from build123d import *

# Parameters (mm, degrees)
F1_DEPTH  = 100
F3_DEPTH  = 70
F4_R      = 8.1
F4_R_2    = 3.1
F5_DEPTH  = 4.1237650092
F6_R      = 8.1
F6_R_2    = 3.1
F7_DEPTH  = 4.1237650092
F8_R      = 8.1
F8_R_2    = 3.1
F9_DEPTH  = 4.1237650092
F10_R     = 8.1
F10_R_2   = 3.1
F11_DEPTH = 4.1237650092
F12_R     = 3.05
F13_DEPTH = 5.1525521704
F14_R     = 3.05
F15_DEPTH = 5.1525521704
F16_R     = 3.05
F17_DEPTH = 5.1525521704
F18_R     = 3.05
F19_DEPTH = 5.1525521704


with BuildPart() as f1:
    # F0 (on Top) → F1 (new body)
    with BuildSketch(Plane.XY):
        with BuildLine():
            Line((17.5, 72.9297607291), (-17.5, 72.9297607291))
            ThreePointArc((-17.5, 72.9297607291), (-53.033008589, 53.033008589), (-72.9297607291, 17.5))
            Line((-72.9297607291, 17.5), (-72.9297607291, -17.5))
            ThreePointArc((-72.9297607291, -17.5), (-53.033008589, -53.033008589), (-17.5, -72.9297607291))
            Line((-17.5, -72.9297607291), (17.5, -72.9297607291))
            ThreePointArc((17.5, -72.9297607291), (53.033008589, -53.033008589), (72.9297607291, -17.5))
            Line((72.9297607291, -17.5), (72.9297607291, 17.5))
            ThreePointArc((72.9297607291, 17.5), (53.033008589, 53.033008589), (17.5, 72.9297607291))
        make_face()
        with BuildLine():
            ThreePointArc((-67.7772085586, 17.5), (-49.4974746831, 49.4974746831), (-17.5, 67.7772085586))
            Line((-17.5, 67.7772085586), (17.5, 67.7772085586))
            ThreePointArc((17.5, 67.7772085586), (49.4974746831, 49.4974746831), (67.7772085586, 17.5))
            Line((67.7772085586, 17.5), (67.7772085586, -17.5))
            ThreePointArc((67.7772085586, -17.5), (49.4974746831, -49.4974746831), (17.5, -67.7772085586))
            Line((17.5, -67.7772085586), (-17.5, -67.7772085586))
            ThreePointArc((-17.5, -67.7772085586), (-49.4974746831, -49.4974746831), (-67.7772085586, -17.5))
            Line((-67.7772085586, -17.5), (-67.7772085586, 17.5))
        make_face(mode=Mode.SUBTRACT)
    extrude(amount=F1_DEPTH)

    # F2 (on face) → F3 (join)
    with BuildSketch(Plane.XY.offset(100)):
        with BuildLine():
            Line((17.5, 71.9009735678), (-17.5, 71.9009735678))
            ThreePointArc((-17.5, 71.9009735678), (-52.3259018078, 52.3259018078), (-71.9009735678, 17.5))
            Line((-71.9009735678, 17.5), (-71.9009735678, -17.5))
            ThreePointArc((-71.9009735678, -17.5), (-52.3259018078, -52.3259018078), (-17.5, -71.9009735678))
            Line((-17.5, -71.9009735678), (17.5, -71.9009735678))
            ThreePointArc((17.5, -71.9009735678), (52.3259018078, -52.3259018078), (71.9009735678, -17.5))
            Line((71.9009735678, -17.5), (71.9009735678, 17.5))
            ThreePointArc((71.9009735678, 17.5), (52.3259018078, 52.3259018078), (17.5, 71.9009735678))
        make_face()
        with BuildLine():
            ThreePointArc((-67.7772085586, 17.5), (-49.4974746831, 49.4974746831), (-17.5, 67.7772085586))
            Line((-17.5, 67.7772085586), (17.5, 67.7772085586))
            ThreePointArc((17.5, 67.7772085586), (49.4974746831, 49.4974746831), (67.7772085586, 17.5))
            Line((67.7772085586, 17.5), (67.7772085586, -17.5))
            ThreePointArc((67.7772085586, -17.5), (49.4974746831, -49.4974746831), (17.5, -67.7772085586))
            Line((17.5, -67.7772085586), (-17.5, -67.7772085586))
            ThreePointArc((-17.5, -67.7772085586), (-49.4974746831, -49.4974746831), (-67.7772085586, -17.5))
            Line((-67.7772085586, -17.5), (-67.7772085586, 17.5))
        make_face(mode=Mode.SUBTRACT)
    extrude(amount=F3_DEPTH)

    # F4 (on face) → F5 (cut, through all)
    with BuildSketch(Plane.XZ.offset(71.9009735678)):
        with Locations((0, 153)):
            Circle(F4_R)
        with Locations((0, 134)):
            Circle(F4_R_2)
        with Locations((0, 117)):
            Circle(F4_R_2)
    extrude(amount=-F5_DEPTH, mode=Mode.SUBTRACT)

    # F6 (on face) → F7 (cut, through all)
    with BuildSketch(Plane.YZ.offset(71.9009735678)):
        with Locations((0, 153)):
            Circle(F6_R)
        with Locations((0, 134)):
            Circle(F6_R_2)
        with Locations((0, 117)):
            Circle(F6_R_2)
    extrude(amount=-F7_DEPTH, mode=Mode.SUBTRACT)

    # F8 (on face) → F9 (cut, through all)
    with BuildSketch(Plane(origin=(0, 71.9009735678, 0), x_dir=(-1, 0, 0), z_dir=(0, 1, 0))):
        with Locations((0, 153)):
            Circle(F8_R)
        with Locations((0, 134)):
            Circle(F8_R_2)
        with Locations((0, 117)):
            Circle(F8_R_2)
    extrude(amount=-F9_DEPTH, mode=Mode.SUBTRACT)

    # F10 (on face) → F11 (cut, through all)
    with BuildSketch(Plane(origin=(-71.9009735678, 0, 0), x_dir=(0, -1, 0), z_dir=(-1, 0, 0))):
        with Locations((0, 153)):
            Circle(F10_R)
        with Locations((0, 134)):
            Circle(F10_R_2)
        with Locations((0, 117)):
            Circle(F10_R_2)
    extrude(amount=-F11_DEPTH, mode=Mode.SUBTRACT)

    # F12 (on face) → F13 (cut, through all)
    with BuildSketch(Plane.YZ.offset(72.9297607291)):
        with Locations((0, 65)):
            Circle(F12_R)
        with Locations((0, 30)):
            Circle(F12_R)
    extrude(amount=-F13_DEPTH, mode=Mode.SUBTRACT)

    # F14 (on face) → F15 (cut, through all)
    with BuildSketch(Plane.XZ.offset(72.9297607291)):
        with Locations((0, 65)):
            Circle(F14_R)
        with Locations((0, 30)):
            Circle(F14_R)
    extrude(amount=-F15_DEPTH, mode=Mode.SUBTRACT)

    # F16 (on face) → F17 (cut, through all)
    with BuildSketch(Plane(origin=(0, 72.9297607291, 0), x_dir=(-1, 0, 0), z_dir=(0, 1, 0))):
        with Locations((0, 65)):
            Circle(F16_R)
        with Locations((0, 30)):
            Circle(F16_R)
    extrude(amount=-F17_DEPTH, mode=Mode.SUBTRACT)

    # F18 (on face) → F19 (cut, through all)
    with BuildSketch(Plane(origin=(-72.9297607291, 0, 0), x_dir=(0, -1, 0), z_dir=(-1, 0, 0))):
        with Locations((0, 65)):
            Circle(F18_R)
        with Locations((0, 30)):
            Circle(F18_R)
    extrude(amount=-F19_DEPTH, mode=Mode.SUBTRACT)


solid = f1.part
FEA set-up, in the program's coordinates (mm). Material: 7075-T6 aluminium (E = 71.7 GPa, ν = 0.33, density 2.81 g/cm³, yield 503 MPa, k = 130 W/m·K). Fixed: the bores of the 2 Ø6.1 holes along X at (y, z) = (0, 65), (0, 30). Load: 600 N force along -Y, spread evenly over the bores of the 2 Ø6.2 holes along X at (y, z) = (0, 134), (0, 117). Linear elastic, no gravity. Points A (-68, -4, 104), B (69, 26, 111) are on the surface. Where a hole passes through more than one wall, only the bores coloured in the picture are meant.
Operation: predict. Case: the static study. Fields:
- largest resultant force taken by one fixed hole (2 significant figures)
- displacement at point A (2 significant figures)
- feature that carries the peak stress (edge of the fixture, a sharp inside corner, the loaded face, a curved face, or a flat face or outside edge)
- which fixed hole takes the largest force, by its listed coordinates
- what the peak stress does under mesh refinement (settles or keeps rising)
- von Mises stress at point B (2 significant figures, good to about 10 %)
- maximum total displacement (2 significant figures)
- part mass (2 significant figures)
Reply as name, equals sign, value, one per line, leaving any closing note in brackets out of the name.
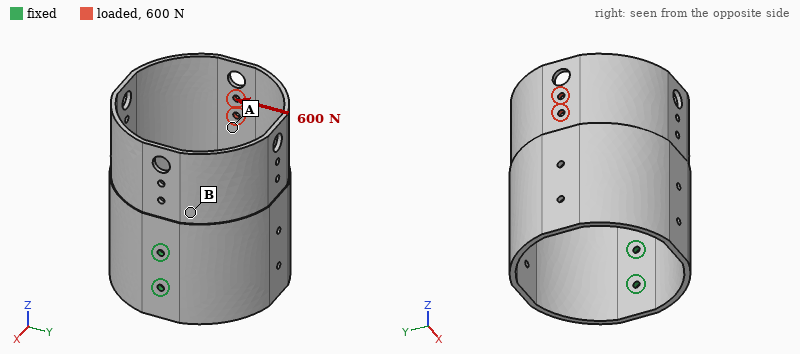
largest resultant force taken by one fixed hole = 1.5 kN
displacement at point A = 2.8 mm
feature that carries the peak stress = edge of the fixture
which fixed hole takes the largest force, by its listed coordinates = (0, 65)
what the peak stress does under mesh refinement = keeps rising
von Mises stress at point B = 29 MPa
maximum total displacement = 2.9 mm
part mass = 990 g
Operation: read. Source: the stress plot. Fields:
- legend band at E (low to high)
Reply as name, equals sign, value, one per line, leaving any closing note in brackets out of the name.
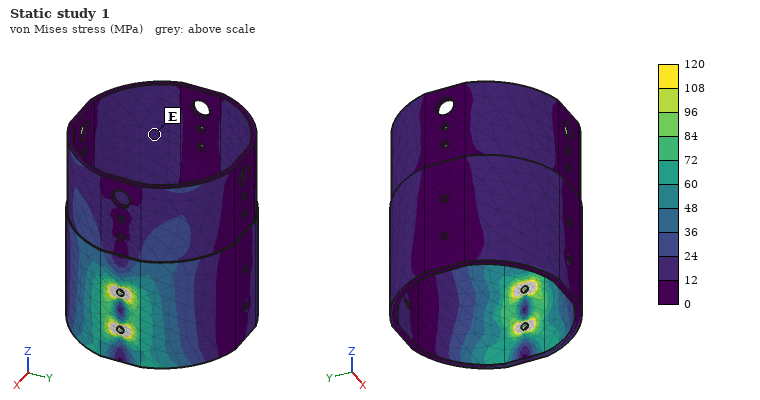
legend band at E = 12 to 24 MPa
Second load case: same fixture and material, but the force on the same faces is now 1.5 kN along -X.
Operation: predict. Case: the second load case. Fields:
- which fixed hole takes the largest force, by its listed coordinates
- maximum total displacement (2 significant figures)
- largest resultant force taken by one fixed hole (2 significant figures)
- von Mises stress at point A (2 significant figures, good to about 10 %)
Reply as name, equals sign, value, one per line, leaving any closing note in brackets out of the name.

which fixed hole takes the largest force, by its listed coordinates = (0, 65)
maximum total displacement = 2.6 mm
largest resultant force taken by one fixed hole = 3.3 kN
von Mises stress at point A = 81 MPa
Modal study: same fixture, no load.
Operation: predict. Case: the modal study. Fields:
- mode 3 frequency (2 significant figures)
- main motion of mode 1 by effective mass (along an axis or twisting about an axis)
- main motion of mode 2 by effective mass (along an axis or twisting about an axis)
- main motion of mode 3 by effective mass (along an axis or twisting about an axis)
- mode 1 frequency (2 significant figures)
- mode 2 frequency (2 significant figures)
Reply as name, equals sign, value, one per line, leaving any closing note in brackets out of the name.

mode 3 frequency = 360 Hz
main motion of mode 1 by effective mass = along Y
main motion of mode 2 by effective mass = along Z
main motion of mode 3 by effective mass = along X
mode 1 frequency = 110 Hz
mode 2 frequency = 190 Hz
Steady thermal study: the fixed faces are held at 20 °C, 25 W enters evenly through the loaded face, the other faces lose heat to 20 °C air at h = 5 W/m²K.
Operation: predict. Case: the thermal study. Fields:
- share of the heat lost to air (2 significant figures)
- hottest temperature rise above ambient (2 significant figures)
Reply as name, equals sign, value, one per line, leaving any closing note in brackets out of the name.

share of the heat lost to air = 43 %
hottest temperature rise above ambient = 40 K
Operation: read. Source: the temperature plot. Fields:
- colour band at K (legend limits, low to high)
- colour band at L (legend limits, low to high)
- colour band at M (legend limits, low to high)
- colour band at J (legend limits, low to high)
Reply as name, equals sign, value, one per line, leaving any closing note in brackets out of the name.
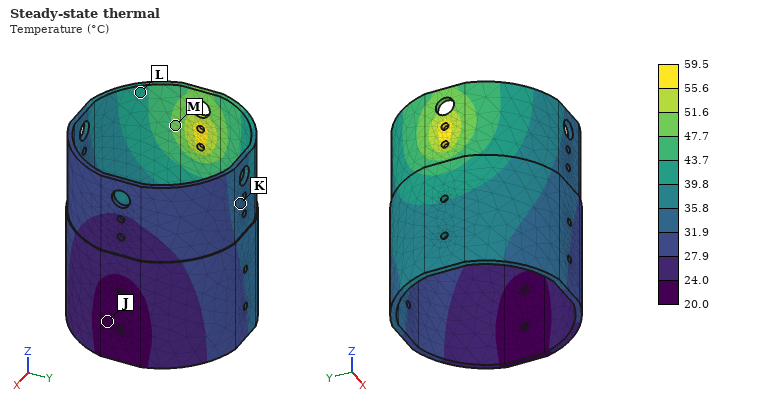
colour band at K = 31.9 to 35.8 °C
colour band at L = 39.8 to 43.7 °C
colour band at M = 47.7 to 51.6 °C
colour band at J = 20.0 to 24.0 °C
